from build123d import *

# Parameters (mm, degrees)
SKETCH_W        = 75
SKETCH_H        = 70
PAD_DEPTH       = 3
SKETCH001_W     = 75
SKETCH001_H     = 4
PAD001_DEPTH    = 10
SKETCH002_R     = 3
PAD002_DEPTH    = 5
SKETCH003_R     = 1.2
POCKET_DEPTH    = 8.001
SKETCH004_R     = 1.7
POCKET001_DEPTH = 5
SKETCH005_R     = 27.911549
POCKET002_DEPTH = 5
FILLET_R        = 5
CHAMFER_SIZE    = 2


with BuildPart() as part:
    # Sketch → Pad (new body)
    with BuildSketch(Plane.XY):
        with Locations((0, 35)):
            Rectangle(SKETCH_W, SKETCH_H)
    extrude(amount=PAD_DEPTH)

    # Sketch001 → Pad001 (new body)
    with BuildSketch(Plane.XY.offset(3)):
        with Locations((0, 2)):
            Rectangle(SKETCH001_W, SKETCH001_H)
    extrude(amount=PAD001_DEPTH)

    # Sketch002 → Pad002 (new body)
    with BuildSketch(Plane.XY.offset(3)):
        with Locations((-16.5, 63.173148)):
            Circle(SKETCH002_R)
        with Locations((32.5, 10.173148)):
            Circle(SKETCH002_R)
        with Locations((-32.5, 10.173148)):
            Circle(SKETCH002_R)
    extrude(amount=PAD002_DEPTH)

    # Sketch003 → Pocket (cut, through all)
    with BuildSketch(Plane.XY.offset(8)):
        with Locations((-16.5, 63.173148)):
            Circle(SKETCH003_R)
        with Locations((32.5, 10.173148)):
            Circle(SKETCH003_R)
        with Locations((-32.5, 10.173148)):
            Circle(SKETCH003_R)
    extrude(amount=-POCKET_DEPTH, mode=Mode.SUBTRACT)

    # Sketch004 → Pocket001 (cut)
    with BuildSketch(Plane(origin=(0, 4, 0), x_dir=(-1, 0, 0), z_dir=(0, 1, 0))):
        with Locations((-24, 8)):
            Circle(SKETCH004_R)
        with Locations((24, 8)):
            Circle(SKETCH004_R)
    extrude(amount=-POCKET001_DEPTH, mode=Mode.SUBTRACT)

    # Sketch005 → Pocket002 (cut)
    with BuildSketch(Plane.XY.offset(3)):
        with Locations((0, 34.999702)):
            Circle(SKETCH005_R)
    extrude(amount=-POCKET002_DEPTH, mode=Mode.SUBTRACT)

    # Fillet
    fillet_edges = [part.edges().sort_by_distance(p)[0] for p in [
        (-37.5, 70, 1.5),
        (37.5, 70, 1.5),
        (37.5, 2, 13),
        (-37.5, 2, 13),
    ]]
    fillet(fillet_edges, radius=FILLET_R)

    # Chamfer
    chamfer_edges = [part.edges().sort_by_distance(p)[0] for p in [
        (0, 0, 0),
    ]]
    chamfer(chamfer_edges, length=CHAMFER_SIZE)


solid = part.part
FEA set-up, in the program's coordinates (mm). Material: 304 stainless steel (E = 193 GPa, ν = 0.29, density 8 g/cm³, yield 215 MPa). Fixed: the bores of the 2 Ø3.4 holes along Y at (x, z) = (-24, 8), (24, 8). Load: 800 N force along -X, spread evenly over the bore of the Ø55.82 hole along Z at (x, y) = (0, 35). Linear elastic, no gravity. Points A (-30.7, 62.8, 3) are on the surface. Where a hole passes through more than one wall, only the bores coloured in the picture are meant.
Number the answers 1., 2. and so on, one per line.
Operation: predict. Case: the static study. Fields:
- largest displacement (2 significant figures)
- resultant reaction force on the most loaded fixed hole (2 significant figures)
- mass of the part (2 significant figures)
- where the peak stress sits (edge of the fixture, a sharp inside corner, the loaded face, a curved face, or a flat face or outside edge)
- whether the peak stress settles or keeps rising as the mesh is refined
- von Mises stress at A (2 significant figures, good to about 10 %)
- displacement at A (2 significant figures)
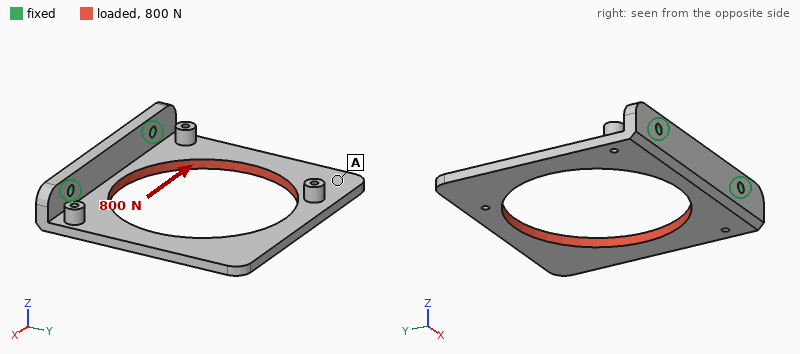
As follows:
1. 70 µm
2. 600 N
3. 91 g
4. edge of the fixture
5. keeps rising
6. 10 MPa
7. 65 µm
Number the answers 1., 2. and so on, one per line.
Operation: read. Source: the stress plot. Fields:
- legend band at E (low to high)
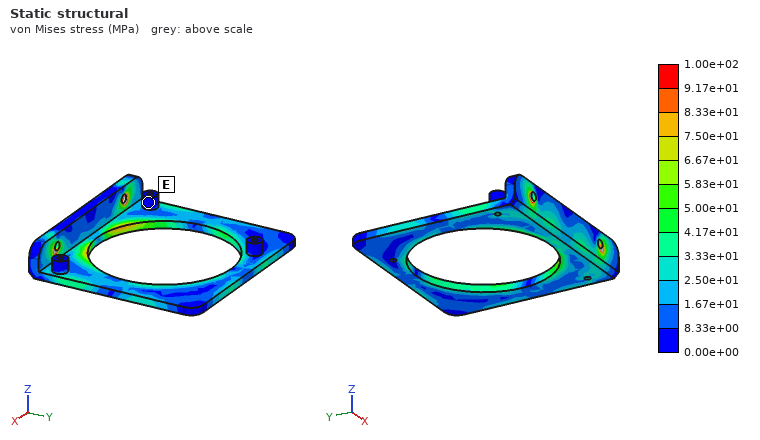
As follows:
1. 0.00e+00 to 8.33e+00 MPa
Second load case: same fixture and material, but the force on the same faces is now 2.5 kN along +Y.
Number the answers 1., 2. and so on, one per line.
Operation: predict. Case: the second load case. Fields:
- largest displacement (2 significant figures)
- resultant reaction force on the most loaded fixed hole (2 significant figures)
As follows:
1. 0.12 mm
2. 1.3 kN
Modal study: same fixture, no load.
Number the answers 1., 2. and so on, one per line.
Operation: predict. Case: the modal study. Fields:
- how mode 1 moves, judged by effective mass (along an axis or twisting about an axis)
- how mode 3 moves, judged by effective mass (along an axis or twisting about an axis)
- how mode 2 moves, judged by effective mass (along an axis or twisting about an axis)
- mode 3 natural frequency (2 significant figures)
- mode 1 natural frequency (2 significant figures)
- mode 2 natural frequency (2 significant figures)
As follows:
1. along Z
2. along X
3. twisting about Y
4. 2300 Hz
5. 390 Hz
6. 880 Hz
